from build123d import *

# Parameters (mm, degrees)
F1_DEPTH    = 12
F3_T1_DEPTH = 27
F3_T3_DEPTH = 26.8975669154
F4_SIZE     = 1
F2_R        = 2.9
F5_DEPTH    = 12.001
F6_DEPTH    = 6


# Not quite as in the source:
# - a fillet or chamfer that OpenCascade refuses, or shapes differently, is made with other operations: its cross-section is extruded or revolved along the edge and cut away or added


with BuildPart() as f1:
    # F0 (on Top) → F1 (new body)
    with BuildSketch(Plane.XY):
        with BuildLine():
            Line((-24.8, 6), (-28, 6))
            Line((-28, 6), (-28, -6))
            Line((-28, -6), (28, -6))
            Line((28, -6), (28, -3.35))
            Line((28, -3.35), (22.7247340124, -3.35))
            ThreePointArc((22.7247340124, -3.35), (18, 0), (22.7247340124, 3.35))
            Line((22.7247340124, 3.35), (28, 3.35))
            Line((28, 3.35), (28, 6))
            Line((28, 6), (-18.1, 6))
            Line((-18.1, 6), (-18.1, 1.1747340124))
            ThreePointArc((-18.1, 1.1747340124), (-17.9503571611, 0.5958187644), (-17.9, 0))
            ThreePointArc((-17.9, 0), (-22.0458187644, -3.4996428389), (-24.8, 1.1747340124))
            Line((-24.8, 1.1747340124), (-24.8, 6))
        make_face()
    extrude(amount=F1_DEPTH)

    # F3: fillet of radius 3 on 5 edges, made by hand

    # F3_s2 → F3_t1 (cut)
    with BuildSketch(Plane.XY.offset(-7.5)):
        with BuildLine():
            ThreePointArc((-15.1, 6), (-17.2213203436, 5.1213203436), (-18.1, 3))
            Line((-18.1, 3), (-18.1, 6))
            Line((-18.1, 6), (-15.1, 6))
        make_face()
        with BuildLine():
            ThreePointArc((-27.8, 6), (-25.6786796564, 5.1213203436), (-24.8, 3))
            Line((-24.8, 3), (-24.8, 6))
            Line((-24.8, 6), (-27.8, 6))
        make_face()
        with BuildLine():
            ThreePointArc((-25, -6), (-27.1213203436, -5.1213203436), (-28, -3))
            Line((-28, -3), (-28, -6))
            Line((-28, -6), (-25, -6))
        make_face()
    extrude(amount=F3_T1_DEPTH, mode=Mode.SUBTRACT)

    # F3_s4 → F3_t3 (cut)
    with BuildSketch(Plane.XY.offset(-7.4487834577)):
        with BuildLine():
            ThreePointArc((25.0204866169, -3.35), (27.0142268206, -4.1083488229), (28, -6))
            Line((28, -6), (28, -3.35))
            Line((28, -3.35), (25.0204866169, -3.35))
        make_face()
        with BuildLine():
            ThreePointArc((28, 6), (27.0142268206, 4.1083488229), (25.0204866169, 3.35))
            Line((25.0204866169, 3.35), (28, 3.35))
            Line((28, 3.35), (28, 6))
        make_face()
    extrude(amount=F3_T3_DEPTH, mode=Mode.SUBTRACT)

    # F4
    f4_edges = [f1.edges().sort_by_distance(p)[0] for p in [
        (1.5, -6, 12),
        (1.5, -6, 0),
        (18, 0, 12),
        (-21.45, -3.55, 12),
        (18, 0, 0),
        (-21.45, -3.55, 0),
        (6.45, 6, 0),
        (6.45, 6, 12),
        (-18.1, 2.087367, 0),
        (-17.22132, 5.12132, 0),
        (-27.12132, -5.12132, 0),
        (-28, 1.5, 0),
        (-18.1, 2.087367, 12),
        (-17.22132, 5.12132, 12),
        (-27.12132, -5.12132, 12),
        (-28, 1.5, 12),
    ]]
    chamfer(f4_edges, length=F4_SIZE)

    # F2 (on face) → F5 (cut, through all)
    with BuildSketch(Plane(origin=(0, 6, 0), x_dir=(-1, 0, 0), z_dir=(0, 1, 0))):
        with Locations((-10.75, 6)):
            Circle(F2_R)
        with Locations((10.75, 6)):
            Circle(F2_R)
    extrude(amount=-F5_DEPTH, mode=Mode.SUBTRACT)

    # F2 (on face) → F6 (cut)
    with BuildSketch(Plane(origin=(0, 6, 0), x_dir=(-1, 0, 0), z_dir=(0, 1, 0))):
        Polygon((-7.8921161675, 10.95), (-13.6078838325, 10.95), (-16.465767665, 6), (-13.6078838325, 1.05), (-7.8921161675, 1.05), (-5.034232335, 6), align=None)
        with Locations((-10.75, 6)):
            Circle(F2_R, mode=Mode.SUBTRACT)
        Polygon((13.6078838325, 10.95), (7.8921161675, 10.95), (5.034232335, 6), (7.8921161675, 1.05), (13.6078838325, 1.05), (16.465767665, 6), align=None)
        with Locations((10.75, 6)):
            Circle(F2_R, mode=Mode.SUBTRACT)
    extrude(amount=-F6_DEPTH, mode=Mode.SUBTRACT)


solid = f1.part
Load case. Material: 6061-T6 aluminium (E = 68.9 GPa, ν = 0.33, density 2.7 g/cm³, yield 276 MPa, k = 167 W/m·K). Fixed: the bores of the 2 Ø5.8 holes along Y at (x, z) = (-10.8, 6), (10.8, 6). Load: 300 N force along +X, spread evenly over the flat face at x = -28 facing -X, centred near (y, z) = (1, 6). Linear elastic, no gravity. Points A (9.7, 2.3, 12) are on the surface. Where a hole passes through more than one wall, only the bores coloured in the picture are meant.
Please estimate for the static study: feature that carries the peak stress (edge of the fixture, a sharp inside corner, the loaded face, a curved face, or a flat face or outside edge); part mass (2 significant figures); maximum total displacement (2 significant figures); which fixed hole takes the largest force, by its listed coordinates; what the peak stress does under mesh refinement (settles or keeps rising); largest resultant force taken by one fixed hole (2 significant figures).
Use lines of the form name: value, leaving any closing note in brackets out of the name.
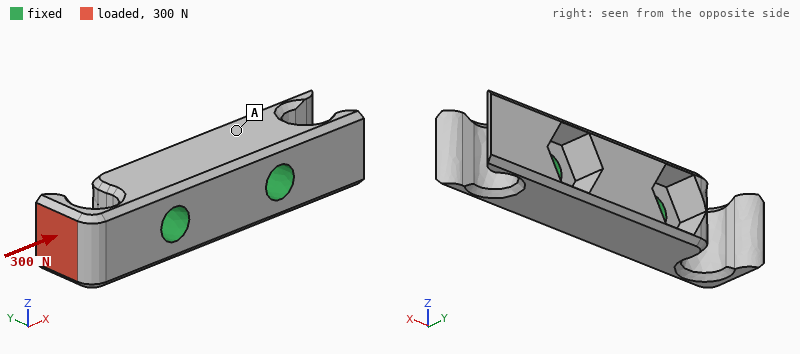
feature that carries the peak stress: a sharp inside corner
part mass: 13 g
maximum total displacement: 0.14 mm
which fixed hole takes the largest force, by its listed coordinates: (-10.8, 6)
what the peak stress does under mesh refinement: keeps rising
largest resultant force taken by one fixed hole: 270 N
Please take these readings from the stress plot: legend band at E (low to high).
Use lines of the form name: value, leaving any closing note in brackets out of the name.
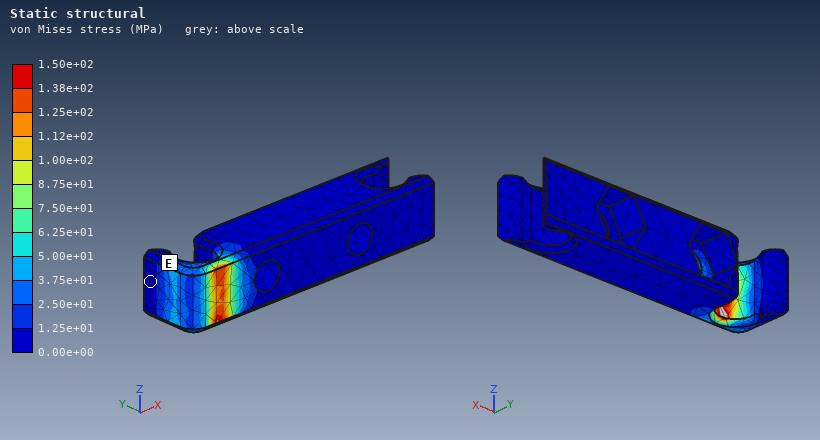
legend band at E: 0.00e+00 to 1.25e+01 MPa
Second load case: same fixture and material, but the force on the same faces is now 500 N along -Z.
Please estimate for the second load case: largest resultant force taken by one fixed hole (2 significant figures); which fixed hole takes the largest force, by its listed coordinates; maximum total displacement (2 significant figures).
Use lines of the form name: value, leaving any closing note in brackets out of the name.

largest resultant force taken by one fixed hole: 590 N
which fixed hole takes the largest force, by its listed coordinates: (-10.8, 6)
maximum total displacement: 0.12 mm
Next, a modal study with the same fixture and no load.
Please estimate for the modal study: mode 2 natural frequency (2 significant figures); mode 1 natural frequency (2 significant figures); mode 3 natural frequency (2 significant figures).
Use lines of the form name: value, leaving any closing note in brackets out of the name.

mode 2 natural frequency: 12 kHz
mode 1 natural frequency: 8000 Hz
mode 3 natural frequency: 18 kHz
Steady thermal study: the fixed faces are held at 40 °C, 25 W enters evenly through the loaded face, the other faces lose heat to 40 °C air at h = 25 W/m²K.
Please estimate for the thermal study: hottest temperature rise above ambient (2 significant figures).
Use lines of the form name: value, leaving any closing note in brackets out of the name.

hottest temperature rise above ambient: 69 K
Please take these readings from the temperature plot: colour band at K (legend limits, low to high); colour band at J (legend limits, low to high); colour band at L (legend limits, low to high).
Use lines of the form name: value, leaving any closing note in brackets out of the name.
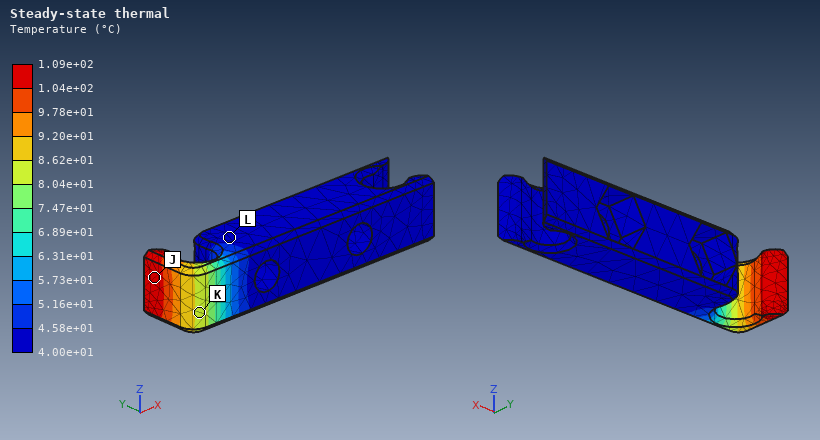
colour band at K: 8.04e+01 to 8.62e+01 °C
colour band at J: 1.04e+02 to 1.09e+02 °C
colour band at L: 4.00e+01 to 4.58e+01 °C
